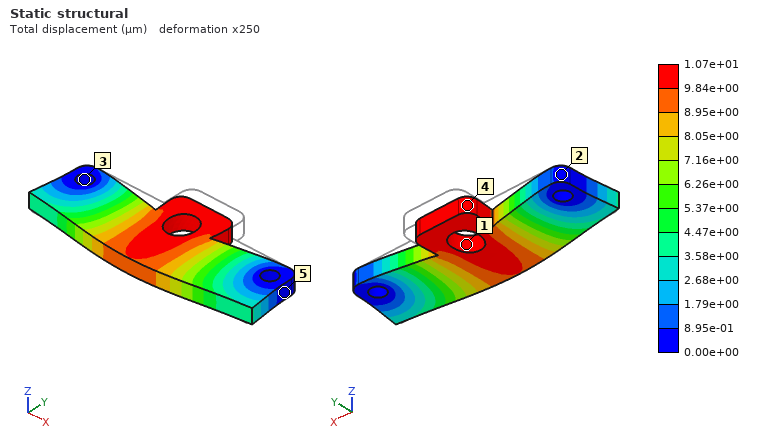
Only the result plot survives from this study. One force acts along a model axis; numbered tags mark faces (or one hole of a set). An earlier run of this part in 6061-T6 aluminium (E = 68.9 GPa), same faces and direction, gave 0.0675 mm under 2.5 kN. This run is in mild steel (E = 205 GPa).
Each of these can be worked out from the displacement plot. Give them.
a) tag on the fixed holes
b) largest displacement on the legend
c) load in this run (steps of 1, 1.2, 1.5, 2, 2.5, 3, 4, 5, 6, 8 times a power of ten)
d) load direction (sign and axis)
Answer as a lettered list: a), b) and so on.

a) 3
b) 1.07e+01 µm
c) 1.2 kN
d) -Y
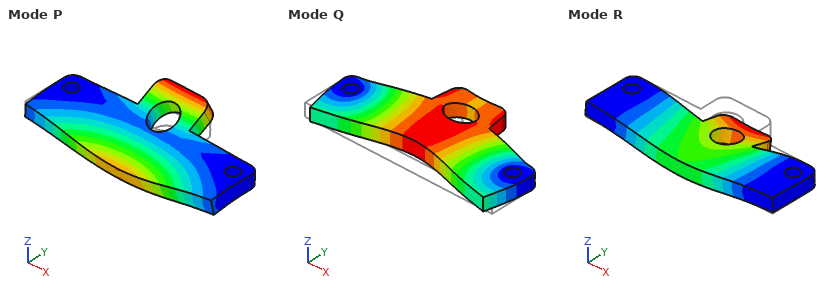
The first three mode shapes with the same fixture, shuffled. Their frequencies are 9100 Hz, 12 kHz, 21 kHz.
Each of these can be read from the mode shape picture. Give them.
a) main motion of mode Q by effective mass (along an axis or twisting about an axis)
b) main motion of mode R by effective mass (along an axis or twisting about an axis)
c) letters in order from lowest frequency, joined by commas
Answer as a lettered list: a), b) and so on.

a) along Y
b) along Z
c) R, P, Q
